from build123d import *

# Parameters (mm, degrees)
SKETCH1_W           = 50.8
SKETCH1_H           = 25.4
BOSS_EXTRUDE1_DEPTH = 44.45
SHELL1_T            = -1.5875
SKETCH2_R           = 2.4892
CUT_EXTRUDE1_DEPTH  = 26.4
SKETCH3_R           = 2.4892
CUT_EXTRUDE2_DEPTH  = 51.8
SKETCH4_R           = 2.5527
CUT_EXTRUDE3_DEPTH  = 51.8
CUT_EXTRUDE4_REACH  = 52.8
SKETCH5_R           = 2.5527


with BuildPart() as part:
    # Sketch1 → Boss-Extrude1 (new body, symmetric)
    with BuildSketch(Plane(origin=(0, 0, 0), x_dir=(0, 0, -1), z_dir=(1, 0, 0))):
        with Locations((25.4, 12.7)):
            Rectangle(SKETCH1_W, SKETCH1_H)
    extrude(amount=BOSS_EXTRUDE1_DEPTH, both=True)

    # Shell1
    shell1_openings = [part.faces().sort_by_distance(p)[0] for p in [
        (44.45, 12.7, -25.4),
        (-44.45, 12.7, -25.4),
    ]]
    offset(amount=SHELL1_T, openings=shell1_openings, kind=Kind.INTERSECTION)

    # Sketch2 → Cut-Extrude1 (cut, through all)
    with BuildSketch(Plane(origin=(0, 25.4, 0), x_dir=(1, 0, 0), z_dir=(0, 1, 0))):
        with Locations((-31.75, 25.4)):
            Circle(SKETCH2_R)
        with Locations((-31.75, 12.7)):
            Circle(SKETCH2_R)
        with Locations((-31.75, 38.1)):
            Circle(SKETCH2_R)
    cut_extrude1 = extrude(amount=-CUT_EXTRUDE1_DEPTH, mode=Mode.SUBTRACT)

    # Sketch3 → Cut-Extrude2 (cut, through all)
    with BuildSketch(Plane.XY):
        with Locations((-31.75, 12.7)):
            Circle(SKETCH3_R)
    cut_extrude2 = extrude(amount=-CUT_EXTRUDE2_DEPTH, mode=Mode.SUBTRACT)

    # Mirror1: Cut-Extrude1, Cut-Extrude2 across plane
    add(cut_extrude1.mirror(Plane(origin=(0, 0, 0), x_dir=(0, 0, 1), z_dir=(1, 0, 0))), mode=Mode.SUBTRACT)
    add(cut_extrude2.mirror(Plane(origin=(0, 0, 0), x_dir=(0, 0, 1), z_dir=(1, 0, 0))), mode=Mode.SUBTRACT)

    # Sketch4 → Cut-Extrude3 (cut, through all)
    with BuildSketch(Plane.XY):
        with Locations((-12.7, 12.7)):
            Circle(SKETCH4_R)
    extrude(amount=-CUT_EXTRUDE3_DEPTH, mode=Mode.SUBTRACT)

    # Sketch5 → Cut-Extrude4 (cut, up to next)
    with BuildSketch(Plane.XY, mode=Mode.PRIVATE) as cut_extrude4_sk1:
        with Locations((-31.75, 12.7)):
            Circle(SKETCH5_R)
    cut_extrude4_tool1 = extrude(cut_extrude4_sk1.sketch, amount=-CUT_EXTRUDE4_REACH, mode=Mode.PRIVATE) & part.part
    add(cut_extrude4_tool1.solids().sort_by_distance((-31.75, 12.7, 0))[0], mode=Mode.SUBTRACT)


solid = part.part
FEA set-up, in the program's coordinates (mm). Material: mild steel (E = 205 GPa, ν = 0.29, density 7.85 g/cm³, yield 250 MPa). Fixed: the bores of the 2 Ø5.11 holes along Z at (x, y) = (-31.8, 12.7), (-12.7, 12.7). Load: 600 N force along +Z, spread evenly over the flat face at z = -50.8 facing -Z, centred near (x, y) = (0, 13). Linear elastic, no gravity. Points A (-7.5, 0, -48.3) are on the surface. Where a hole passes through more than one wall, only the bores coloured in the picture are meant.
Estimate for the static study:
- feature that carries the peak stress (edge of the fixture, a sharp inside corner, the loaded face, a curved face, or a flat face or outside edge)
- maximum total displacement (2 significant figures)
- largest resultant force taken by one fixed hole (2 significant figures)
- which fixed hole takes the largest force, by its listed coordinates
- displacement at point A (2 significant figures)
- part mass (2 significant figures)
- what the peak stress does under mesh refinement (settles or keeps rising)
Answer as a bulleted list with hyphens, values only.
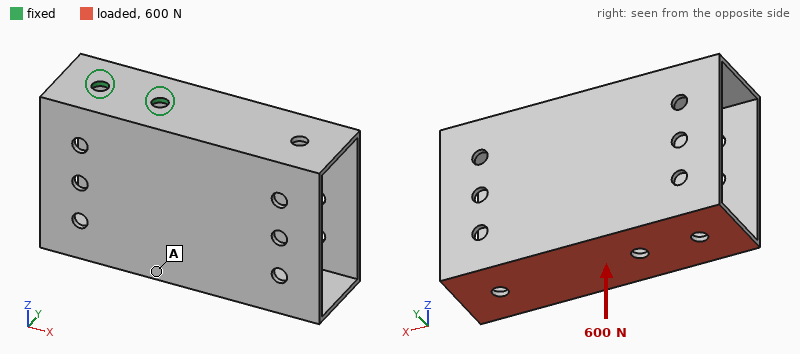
- edge of the fixture
- 0.27 mm
- 820 N
- (-12.7, 12.7)
- 0.15 mm
- 160 g
- keeps rising
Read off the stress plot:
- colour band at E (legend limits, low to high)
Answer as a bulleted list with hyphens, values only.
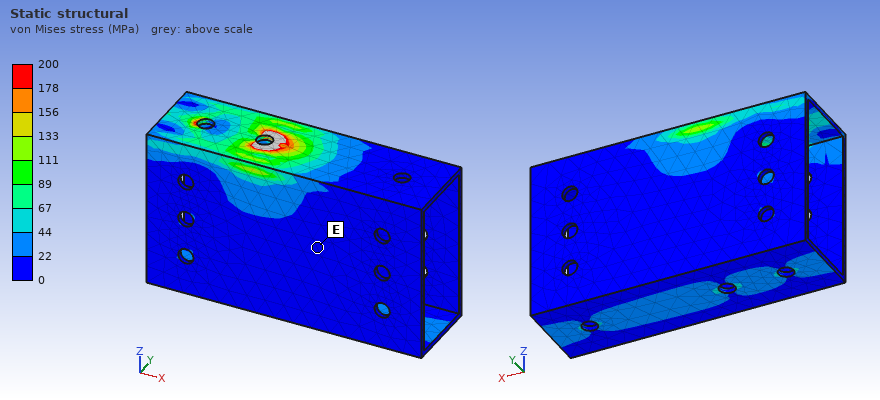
- 0 to 22 MPa
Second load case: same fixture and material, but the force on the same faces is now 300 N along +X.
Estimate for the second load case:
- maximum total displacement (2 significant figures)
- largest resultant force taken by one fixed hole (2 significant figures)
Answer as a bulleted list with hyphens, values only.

- 0.29 mm
- 610 N
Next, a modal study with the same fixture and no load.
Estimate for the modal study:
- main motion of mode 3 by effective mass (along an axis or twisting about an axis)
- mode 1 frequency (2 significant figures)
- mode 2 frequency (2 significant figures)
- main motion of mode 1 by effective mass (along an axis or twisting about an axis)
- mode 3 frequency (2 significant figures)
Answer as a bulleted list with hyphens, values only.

- twisting about Z
- 360 Hz
- 580 Hz
- along Y
- 1200 Hz
